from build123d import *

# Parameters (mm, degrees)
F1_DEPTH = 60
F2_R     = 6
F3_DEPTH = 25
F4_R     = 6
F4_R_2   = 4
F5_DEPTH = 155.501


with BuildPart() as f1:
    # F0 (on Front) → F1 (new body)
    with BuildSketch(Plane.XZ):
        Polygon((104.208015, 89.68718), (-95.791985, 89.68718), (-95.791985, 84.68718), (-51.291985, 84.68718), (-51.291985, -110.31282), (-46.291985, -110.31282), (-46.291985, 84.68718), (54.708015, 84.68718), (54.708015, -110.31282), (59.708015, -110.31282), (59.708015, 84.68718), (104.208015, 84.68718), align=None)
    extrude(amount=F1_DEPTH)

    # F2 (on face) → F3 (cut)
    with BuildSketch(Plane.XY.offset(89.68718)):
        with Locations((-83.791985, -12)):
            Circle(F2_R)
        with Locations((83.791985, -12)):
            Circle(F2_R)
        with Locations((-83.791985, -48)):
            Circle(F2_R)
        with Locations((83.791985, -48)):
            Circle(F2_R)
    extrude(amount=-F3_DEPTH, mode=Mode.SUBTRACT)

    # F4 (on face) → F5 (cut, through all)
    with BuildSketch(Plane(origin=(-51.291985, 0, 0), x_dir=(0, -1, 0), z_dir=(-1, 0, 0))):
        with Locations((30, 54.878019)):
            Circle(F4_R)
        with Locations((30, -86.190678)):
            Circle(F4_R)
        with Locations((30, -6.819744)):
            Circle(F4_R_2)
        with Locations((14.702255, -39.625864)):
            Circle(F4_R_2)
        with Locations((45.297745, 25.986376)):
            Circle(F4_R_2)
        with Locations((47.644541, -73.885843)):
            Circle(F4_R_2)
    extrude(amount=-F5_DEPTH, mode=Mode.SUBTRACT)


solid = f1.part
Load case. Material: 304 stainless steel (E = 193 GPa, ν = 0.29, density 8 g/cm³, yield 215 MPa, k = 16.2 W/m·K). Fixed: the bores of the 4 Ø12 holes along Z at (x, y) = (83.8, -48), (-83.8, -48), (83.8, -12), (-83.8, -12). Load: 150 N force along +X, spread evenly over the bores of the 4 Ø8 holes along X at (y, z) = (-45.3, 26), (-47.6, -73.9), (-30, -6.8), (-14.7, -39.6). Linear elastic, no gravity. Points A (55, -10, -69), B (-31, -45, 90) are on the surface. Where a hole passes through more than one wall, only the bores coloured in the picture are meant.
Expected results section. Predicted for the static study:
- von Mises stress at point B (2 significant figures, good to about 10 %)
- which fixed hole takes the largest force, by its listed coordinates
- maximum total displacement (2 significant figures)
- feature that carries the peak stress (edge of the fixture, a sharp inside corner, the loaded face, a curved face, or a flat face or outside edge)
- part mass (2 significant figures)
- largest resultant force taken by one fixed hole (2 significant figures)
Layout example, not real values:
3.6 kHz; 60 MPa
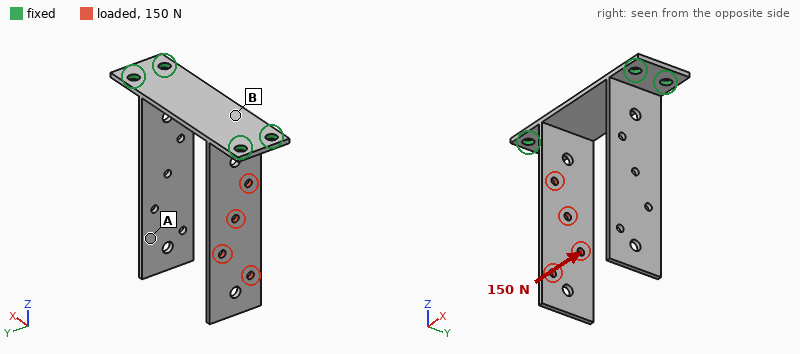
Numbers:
22 MPa; (-83.8, -48); 1.6 mm; a curved face; 1.4 kg; 92 N
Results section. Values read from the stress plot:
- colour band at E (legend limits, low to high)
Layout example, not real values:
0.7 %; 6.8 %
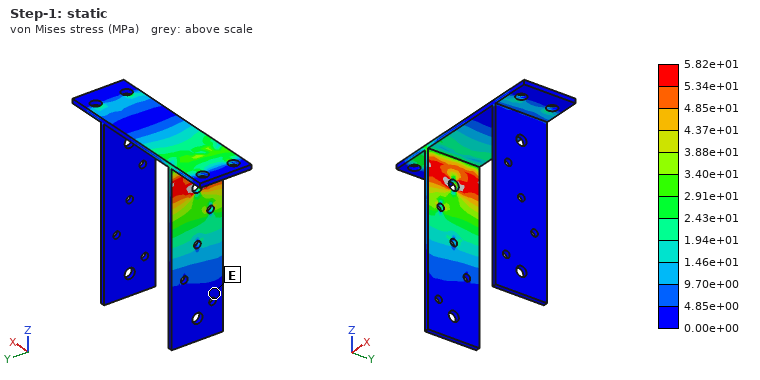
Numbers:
0.00e+00 to 4.85e+00 MPa
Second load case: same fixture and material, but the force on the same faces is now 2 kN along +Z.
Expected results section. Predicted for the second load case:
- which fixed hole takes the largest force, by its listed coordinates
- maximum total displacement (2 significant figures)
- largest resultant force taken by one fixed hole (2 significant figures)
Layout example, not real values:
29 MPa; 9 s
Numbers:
(-83.8, -48); 0.62 mm; 1.1 kN
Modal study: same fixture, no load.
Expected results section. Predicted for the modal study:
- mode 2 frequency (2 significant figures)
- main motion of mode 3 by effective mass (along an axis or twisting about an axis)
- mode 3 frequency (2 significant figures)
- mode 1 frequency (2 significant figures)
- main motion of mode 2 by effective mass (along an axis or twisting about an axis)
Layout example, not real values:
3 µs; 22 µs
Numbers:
97 Hz; along Y; 270 Hz; 90 Hz; along X
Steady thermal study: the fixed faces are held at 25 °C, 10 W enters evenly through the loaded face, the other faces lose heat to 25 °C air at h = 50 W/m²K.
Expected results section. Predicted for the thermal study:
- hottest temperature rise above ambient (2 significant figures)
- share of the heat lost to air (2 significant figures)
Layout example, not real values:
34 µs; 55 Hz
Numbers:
18 K; 99 %
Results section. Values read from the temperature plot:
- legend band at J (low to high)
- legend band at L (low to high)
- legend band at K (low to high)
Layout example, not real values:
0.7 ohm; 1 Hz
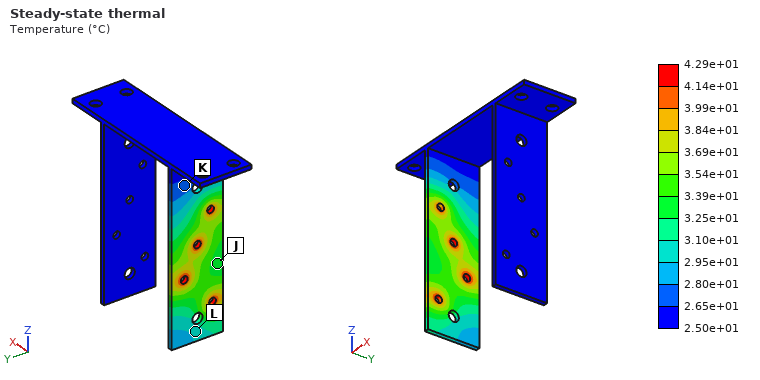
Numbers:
3.25e+01 to 3.39e+01 °C; 2.95e+01 to 3.10e+01 °C; 2.65e+01 to 2.80e+01 °C
